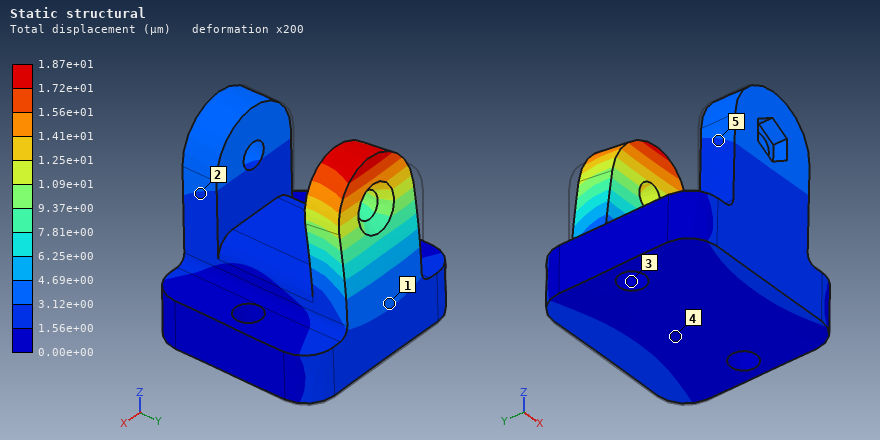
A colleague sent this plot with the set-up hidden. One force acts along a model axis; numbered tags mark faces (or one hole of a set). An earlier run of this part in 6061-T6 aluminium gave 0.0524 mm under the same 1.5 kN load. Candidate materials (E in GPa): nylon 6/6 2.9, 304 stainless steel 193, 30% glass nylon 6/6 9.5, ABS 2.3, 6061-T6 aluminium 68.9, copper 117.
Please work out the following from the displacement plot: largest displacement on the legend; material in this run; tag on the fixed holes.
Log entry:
1.87e+01 µm
304 stainless steel
3
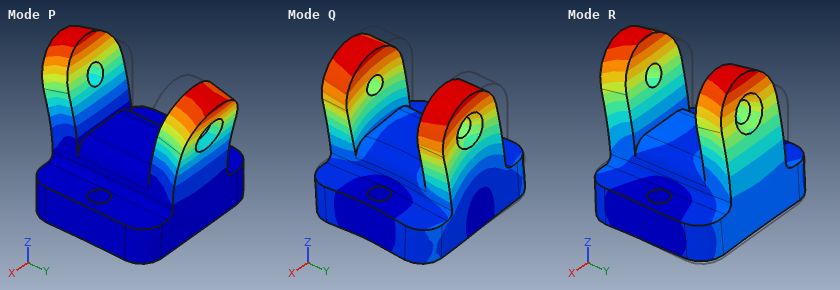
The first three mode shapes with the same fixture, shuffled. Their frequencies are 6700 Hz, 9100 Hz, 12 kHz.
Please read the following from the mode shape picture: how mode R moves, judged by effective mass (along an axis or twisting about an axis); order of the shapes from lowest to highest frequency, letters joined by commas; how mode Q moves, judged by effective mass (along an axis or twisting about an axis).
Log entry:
along Y
R, P, Q
along X
